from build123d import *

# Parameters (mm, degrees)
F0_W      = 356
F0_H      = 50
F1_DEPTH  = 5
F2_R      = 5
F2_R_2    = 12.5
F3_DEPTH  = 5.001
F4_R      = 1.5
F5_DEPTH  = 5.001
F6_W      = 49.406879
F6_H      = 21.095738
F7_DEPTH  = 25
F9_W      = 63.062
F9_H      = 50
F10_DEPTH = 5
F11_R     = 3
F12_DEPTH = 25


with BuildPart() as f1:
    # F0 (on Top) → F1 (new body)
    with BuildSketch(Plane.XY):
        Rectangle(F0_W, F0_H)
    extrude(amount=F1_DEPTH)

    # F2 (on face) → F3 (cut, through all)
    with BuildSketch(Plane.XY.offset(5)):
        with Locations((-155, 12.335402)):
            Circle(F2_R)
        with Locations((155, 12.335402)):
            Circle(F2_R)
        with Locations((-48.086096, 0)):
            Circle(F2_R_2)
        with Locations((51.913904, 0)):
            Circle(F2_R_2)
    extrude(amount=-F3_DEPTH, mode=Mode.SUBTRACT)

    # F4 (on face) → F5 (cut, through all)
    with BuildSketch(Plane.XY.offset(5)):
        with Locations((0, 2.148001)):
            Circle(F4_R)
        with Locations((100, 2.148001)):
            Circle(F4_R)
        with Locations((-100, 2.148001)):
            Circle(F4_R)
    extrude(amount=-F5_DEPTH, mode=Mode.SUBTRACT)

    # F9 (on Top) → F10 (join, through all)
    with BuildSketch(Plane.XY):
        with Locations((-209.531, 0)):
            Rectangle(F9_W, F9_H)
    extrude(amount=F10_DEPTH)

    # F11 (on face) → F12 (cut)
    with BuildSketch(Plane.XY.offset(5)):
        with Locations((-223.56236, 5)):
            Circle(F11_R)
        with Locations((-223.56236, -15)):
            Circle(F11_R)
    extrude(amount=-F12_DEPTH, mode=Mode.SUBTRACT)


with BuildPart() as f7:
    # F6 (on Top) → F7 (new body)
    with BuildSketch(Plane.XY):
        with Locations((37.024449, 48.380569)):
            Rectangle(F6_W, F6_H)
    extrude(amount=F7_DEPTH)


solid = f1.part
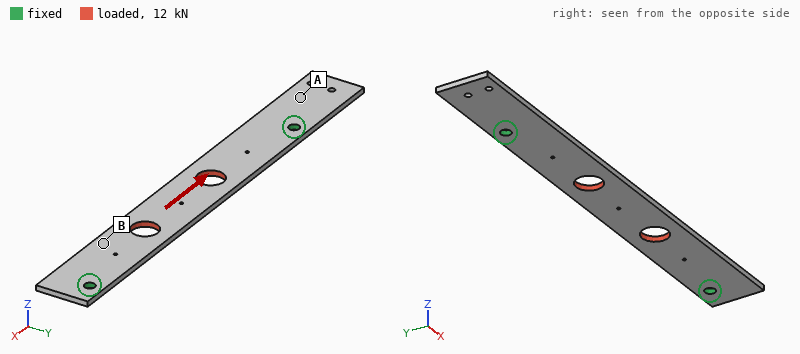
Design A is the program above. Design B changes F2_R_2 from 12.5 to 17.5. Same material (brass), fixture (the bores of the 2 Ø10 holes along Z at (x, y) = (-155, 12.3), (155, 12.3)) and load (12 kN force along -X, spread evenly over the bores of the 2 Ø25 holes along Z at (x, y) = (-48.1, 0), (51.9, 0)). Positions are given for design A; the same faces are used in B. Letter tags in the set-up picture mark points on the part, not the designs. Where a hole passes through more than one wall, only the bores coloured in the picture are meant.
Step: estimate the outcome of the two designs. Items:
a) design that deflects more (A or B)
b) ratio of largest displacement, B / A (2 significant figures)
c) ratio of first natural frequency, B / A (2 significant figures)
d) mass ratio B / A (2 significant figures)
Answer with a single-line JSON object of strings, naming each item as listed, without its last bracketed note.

{"design that deflects more": "B", "ratio of largest displacement, B / A": "1.1", "ratio of first natural frequency, B / A": "1.0", "mass ratio B / A": "0.95"}
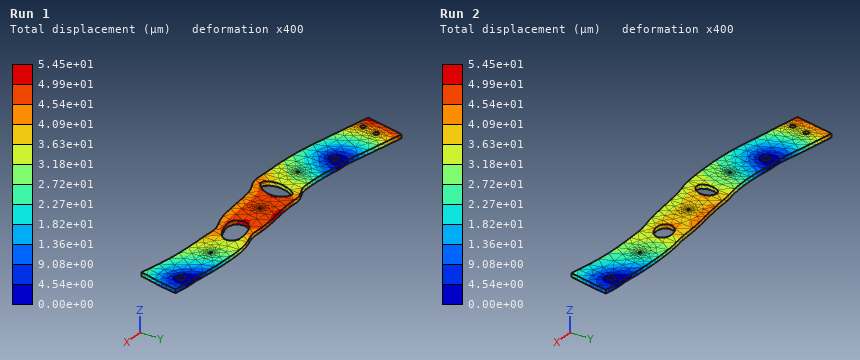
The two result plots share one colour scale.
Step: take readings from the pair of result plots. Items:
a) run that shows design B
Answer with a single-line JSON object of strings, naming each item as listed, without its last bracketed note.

{"run that shows design B": "Run 1"}
